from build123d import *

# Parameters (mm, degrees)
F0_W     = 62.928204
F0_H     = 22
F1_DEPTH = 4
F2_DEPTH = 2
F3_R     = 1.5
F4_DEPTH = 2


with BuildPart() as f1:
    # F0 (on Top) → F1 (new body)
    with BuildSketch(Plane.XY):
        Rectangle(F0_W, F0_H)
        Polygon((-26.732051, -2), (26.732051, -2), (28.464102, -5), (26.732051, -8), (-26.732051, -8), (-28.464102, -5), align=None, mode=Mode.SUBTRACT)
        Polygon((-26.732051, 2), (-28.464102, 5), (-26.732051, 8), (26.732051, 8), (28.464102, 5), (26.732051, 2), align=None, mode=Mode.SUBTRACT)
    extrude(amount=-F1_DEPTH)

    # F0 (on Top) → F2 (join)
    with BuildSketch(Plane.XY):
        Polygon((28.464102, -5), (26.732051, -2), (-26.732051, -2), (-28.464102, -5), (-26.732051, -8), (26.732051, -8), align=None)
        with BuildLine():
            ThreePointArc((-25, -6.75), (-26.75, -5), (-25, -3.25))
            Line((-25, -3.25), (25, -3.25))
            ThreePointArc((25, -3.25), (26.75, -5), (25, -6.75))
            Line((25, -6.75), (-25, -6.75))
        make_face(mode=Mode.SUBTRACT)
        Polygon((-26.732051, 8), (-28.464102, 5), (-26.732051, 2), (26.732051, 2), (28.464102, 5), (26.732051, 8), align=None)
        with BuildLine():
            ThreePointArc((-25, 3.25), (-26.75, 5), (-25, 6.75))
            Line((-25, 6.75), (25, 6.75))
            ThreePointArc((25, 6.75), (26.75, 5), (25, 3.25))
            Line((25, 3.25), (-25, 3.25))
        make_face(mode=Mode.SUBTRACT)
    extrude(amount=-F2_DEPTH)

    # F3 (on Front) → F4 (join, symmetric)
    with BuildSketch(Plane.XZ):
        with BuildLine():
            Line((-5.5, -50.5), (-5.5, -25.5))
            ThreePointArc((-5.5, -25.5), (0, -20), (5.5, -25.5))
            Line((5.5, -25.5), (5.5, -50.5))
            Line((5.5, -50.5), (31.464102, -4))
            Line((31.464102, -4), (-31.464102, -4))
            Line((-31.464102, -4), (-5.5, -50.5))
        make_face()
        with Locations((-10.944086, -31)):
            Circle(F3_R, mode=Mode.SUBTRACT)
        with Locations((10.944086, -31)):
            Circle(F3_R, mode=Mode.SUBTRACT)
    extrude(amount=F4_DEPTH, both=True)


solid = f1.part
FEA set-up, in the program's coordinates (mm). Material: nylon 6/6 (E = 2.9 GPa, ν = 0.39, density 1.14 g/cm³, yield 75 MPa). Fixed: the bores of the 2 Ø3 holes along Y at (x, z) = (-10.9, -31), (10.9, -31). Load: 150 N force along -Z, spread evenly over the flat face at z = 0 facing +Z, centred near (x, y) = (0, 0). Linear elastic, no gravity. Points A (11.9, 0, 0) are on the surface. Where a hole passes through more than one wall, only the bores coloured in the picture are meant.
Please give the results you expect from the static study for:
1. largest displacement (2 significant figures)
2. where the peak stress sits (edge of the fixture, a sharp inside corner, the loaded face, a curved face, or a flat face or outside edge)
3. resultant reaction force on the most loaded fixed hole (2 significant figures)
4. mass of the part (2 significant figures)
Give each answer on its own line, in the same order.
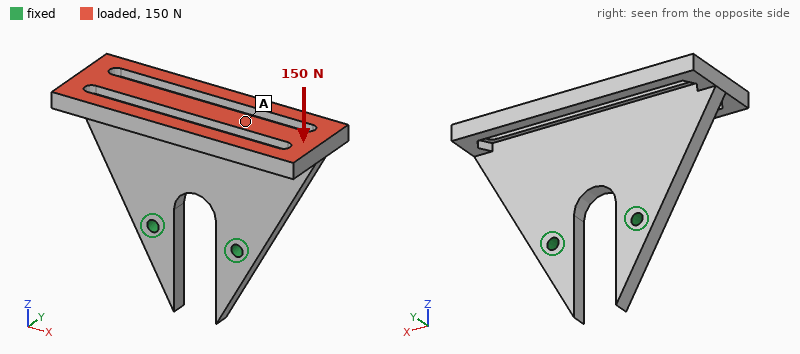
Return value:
0.81 mm
a curved face
78 N
10 g
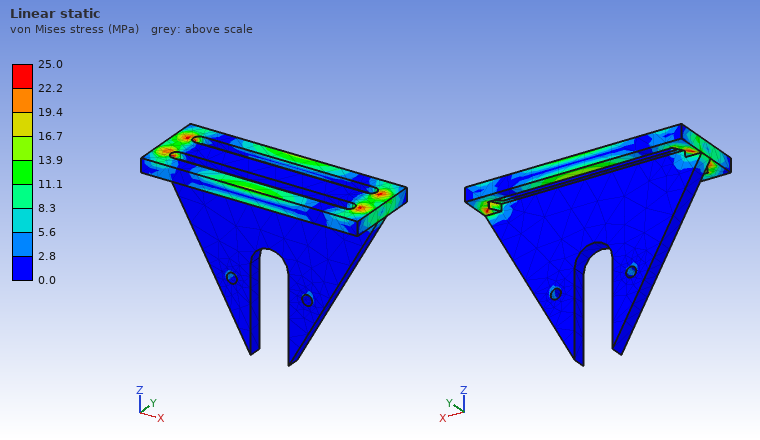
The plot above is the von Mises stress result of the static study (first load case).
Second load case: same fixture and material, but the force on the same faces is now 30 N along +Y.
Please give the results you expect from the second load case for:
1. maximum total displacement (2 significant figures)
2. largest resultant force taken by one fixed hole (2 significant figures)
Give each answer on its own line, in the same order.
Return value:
0.82 mm
15 N
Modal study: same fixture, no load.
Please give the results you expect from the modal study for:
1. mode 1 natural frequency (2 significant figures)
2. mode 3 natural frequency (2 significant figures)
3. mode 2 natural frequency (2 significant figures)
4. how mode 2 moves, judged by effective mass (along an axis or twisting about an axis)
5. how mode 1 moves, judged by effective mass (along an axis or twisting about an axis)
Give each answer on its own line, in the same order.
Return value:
480 Hz
1100 Hz
720 Hz
twisting about Z
along Y
